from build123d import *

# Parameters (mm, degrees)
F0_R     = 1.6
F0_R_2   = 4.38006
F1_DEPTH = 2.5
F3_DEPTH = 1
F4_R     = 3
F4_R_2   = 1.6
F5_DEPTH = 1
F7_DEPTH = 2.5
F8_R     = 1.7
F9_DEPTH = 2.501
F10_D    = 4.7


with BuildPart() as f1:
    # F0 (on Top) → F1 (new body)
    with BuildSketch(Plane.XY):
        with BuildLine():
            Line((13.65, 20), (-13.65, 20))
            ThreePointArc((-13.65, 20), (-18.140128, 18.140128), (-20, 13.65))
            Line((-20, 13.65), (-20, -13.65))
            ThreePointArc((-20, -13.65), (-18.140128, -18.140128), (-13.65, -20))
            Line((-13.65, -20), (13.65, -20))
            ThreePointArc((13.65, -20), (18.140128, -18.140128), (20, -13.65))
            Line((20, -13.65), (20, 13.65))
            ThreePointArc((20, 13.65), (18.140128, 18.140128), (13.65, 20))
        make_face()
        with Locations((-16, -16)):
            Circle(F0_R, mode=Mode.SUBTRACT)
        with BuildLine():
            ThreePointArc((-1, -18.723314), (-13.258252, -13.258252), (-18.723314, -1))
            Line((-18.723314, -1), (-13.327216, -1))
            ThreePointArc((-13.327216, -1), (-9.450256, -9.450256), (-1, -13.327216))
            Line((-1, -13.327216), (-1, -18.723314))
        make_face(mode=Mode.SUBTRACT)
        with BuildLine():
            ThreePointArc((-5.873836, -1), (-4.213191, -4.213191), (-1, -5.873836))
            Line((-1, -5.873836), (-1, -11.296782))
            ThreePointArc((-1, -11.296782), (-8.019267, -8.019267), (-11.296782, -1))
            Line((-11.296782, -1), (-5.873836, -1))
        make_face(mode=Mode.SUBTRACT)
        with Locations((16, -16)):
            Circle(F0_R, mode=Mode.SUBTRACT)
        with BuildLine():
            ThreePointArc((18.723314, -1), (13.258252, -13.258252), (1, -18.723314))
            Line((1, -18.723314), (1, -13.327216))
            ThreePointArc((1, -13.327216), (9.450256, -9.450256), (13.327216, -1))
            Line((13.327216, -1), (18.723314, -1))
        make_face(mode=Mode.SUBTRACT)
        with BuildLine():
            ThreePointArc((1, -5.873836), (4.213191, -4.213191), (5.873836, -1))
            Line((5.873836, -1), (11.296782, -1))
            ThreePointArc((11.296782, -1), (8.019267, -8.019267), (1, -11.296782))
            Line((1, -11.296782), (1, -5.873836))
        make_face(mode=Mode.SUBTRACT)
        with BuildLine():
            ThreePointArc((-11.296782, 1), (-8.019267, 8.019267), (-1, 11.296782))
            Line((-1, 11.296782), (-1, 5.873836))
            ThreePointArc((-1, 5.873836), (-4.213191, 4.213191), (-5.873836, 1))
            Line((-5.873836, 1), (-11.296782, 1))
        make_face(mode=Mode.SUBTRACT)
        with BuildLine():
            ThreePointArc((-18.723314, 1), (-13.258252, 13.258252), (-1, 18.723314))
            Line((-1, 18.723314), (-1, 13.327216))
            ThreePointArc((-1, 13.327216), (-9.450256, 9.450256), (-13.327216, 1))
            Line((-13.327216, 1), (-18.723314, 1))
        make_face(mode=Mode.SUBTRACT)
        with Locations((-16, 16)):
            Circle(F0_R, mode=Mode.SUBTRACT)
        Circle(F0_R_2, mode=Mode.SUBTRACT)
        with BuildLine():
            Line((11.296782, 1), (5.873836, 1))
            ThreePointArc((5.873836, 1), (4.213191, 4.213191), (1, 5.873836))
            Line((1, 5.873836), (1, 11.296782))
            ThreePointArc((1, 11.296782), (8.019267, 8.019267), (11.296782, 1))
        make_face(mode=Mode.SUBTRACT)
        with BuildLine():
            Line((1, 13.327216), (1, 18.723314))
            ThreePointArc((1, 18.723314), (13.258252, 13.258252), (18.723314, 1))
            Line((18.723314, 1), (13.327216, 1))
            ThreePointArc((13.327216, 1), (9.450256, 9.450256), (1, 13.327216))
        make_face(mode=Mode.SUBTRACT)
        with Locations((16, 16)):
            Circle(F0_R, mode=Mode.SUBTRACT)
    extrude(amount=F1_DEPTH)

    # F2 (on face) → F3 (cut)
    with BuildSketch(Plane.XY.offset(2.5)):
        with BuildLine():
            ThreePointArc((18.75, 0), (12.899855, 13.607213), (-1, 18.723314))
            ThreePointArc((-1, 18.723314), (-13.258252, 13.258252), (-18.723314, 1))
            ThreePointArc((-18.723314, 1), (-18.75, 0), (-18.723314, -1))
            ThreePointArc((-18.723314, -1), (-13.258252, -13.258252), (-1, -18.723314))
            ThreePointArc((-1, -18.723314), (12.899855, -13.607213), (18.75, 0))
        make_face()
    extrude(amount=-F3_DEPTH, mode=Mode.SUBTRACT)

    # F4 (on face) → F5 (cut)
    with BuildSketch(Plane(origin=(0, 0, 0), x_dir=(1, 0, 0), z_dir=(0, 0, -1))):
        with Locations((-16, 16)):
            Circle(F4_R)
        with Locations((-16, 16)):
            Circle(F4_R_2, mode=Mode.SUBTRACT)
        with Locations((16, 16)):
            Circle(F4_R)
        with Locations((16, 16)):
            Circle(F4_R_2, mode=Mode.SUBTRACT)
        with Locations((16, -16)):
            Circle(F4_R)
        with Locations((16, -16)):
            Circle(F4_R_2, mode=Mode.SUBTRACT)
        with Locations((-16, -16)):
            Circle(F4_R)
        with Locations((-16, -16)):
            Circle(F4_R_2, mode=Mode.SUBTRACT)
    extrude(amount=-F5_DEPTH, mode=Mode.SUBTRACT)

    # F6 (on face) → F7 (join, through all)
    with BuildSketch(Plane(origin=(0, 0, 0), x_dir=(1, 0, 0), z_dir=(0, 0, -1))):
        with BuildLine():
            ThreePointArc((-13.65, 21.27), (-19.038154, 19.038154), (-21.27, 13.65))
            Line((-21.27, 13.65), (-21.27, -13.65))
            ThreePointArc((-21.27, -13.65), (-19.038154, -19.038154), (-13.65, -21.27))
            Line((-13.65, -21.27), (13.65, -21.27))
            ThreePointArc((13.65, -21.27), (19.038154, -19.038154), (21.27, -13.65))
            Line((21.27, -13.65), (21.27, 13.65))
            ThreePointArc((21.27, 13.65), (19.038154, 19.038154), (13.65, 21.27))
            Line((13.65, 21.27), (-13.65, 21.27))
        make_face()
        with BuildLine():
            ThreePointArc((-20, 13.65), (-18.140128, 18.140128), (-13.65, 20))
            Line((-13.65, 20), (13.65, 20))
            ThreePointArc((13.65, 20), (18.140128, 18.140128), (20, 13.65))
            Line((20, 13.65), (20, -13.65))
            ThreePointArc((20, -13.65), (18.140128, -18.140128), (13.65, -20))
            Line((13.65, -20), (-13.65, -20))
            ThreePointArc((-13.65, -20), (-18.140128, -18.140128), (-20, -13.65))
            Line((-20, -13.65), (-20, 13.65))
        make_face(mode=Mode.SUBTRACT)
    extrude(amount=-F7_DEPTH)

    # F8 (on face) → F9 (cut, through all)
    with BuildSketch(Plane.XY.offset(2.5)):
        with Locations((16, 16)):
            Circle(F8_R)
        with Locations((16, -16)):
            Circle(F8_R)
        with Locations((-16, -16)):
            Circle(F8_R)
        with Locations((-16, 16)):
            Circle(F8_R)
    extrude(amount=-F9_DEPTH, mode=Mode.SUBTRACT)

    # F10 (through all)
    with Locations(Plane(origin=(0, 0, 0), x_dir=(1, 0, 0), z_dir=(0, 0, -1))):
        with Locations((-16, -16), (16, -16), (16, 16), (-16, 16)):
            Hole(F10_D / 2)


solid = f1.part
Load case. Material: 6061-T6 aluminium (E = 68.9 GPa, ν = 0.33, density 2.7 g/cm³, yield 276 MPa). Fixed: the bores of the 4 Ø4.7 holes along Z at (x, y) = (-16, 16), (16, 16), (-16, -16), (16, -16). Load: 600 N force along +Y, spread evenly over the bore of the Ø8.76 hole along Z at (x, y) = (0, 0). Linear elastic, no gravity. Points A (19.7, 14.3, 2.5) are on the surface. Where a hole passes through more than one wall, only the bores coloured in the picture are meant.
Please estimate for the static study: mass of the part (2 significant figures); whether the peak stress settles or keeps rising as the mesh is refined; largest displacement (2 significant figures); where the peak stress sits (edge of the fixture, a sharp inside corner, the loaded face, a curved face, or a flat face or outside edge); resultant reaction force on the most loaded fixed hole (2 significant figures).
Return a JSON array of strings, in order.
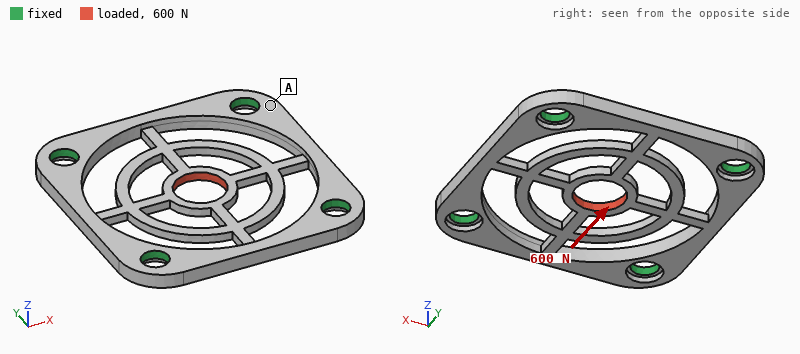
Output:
["5.0 g", "keeps rising", "69 µm", "a sharp inside corner", "210 N"]
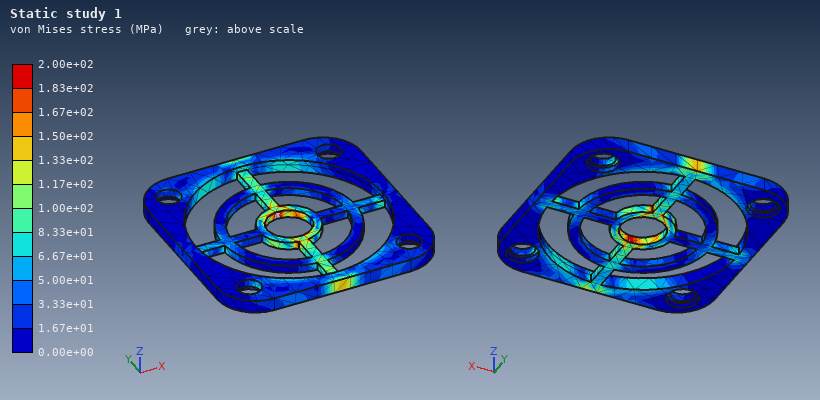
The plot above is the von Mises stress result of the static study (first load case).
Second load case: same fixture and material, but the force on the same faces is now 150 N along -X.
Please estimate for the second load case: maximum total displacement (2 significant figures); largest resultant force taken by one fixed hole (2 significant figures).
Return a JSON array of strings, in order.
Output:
["17 µm", "53 N"]
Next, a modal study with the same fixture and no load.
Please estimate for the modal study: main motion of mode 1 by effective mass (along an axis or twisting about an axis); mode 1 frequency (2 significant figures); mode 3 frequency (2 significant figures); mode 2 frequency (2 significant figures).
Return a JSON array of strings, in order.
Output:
["along Z", "4700 Hz", "7900 Hz", "7900 Hz"]
